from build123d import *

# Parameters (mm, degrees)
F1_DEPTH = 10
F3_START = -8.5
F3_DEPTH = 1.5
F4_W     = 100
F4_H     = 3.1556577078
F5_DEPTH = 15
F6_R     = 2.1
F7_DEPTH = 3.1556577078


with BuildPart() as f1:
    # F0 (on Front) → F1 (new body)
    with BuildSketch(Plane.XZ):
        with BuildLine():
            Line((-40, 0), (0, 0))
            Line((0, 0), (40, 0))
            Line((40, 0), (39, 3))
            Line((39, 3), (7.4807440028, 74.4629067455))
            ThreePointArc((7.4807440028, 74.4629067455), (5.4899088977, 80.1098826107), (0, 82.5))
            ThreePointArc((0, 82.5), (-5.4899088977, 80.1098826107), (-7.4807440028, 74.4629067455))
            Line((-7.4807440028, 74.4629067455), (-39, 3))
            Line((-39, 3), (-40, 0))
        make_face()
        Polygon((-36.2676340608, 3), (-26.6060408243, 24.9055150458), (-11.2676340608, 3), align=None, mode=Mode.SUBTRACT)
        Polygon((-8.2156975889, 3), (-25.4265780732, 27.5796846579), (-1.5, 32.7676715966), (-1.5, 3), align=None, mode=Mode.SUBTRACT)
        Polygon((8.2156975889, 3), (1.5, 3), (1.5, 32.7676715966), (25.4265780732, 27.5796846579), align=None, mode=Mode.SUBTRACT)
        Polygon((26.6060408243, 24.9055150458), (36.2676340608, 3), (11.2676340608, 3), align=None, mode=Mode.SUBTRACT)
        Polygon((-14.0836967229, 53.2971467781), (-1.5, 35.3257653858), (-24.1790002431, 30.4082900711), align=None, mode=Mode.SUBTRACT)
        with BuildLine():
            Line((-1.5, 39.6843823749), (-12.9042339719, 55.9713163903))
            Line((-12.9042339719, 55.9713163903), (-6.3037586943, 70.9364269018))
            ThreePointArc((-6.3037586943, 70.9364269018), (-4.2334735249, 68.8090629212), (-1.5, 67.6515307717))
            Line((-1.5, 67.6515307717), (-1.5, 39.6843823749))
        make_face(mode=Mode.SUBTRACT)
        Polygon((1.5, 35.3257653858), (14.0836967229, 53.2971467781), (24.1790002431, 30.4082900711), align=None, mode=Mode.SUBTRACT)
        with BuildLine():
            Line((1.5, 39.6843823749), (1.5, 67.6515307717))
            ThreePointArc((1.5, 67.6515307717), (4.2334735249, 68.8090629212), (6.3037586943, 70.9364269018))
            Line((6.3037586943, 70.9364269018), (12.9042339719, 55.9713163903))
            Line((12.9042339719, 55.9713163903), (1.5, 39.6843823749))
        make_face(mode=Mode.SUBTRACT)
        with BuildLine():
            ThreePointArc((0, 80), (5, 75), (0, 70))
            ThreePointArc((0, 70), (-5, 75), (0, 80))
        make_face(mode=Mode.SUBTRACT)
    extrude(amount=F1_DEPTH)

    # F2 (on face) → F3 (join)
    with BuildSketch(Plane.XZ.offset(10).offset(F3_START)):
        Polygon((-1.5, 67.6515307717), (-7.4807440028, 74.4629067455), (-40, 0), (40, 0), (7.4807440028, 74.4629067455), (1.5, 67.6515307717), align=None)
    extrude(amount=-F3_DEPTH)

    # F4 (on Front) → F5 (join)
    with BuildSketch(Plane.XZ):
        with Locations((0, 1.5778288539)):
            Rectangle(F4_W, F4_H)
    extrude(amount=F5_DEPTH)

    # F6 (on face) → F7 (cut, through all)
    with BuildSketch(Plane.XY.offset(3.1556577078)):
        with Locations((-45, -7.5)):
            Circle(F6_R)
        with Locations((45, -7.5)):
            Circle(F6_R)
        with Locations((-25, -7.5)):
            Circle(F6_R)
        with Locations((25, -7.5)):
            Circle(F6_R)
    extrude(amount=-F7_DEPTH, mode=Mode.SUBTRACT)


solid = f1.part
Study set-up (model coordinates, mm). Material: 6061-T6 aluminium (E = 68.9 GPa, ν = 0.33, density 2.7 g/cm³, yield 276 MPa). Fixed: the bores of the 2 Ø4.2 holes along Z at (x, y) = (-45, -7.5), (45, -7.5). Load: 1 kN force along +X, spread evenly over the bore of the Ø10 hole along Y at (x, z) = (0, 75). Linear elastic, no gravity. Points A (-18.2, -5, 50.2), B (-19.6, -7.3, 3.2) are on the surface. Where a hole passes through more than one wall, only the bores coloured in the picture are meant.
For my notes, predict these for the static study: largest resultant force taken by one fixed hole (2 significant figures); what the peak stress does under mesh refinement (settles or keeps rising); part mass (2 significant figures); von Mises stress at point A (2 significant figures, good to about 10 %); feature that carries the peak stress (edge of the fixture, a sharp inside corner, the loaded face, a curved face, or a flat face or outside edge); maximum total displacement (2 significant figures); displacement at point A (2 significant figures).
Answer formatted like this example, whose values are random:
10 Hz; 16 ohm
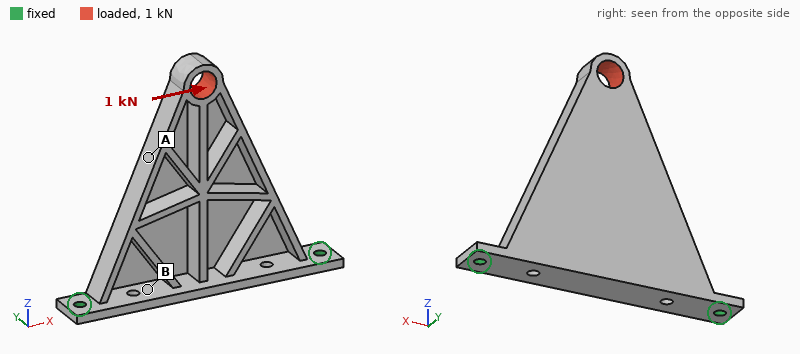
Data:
1.0 kN; keeps rising; 50 g; 31 MPa; edge of the fixture; 0.16 mm; 0.076 mm
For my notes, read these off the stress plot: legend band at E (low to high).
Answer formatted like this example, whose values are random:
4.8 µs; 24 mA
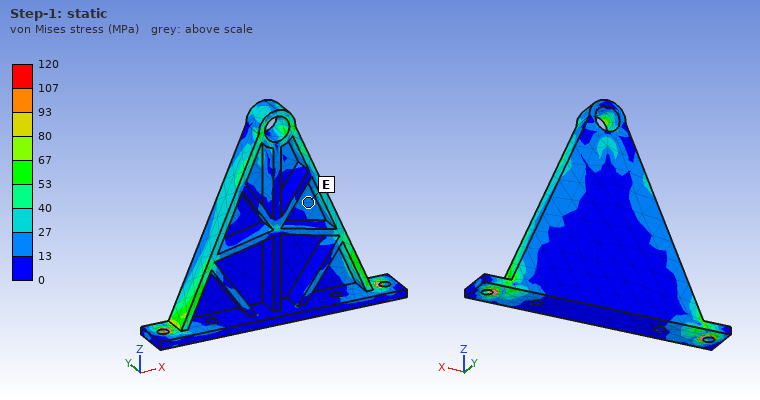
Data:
13 to 27 MPa
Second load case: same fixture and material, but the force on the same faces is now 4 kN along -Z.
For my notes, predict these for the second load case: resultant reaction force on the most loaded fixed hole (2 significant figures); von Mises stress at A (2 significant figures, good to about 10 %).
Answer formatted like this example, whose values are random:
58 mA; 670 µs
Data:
2.3 kN; 46 MPa
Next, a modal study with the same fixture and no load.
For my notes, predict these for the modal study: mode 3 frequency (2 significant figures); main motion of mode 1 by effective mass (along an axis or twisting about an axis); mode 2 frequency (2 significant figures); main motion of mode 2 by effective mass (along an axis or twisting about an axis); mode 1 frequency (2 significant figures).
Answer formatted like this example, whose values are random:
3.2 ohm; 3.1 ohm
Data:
4300 Hz; along Y; 3800 Hz; along X; 620 Hz
